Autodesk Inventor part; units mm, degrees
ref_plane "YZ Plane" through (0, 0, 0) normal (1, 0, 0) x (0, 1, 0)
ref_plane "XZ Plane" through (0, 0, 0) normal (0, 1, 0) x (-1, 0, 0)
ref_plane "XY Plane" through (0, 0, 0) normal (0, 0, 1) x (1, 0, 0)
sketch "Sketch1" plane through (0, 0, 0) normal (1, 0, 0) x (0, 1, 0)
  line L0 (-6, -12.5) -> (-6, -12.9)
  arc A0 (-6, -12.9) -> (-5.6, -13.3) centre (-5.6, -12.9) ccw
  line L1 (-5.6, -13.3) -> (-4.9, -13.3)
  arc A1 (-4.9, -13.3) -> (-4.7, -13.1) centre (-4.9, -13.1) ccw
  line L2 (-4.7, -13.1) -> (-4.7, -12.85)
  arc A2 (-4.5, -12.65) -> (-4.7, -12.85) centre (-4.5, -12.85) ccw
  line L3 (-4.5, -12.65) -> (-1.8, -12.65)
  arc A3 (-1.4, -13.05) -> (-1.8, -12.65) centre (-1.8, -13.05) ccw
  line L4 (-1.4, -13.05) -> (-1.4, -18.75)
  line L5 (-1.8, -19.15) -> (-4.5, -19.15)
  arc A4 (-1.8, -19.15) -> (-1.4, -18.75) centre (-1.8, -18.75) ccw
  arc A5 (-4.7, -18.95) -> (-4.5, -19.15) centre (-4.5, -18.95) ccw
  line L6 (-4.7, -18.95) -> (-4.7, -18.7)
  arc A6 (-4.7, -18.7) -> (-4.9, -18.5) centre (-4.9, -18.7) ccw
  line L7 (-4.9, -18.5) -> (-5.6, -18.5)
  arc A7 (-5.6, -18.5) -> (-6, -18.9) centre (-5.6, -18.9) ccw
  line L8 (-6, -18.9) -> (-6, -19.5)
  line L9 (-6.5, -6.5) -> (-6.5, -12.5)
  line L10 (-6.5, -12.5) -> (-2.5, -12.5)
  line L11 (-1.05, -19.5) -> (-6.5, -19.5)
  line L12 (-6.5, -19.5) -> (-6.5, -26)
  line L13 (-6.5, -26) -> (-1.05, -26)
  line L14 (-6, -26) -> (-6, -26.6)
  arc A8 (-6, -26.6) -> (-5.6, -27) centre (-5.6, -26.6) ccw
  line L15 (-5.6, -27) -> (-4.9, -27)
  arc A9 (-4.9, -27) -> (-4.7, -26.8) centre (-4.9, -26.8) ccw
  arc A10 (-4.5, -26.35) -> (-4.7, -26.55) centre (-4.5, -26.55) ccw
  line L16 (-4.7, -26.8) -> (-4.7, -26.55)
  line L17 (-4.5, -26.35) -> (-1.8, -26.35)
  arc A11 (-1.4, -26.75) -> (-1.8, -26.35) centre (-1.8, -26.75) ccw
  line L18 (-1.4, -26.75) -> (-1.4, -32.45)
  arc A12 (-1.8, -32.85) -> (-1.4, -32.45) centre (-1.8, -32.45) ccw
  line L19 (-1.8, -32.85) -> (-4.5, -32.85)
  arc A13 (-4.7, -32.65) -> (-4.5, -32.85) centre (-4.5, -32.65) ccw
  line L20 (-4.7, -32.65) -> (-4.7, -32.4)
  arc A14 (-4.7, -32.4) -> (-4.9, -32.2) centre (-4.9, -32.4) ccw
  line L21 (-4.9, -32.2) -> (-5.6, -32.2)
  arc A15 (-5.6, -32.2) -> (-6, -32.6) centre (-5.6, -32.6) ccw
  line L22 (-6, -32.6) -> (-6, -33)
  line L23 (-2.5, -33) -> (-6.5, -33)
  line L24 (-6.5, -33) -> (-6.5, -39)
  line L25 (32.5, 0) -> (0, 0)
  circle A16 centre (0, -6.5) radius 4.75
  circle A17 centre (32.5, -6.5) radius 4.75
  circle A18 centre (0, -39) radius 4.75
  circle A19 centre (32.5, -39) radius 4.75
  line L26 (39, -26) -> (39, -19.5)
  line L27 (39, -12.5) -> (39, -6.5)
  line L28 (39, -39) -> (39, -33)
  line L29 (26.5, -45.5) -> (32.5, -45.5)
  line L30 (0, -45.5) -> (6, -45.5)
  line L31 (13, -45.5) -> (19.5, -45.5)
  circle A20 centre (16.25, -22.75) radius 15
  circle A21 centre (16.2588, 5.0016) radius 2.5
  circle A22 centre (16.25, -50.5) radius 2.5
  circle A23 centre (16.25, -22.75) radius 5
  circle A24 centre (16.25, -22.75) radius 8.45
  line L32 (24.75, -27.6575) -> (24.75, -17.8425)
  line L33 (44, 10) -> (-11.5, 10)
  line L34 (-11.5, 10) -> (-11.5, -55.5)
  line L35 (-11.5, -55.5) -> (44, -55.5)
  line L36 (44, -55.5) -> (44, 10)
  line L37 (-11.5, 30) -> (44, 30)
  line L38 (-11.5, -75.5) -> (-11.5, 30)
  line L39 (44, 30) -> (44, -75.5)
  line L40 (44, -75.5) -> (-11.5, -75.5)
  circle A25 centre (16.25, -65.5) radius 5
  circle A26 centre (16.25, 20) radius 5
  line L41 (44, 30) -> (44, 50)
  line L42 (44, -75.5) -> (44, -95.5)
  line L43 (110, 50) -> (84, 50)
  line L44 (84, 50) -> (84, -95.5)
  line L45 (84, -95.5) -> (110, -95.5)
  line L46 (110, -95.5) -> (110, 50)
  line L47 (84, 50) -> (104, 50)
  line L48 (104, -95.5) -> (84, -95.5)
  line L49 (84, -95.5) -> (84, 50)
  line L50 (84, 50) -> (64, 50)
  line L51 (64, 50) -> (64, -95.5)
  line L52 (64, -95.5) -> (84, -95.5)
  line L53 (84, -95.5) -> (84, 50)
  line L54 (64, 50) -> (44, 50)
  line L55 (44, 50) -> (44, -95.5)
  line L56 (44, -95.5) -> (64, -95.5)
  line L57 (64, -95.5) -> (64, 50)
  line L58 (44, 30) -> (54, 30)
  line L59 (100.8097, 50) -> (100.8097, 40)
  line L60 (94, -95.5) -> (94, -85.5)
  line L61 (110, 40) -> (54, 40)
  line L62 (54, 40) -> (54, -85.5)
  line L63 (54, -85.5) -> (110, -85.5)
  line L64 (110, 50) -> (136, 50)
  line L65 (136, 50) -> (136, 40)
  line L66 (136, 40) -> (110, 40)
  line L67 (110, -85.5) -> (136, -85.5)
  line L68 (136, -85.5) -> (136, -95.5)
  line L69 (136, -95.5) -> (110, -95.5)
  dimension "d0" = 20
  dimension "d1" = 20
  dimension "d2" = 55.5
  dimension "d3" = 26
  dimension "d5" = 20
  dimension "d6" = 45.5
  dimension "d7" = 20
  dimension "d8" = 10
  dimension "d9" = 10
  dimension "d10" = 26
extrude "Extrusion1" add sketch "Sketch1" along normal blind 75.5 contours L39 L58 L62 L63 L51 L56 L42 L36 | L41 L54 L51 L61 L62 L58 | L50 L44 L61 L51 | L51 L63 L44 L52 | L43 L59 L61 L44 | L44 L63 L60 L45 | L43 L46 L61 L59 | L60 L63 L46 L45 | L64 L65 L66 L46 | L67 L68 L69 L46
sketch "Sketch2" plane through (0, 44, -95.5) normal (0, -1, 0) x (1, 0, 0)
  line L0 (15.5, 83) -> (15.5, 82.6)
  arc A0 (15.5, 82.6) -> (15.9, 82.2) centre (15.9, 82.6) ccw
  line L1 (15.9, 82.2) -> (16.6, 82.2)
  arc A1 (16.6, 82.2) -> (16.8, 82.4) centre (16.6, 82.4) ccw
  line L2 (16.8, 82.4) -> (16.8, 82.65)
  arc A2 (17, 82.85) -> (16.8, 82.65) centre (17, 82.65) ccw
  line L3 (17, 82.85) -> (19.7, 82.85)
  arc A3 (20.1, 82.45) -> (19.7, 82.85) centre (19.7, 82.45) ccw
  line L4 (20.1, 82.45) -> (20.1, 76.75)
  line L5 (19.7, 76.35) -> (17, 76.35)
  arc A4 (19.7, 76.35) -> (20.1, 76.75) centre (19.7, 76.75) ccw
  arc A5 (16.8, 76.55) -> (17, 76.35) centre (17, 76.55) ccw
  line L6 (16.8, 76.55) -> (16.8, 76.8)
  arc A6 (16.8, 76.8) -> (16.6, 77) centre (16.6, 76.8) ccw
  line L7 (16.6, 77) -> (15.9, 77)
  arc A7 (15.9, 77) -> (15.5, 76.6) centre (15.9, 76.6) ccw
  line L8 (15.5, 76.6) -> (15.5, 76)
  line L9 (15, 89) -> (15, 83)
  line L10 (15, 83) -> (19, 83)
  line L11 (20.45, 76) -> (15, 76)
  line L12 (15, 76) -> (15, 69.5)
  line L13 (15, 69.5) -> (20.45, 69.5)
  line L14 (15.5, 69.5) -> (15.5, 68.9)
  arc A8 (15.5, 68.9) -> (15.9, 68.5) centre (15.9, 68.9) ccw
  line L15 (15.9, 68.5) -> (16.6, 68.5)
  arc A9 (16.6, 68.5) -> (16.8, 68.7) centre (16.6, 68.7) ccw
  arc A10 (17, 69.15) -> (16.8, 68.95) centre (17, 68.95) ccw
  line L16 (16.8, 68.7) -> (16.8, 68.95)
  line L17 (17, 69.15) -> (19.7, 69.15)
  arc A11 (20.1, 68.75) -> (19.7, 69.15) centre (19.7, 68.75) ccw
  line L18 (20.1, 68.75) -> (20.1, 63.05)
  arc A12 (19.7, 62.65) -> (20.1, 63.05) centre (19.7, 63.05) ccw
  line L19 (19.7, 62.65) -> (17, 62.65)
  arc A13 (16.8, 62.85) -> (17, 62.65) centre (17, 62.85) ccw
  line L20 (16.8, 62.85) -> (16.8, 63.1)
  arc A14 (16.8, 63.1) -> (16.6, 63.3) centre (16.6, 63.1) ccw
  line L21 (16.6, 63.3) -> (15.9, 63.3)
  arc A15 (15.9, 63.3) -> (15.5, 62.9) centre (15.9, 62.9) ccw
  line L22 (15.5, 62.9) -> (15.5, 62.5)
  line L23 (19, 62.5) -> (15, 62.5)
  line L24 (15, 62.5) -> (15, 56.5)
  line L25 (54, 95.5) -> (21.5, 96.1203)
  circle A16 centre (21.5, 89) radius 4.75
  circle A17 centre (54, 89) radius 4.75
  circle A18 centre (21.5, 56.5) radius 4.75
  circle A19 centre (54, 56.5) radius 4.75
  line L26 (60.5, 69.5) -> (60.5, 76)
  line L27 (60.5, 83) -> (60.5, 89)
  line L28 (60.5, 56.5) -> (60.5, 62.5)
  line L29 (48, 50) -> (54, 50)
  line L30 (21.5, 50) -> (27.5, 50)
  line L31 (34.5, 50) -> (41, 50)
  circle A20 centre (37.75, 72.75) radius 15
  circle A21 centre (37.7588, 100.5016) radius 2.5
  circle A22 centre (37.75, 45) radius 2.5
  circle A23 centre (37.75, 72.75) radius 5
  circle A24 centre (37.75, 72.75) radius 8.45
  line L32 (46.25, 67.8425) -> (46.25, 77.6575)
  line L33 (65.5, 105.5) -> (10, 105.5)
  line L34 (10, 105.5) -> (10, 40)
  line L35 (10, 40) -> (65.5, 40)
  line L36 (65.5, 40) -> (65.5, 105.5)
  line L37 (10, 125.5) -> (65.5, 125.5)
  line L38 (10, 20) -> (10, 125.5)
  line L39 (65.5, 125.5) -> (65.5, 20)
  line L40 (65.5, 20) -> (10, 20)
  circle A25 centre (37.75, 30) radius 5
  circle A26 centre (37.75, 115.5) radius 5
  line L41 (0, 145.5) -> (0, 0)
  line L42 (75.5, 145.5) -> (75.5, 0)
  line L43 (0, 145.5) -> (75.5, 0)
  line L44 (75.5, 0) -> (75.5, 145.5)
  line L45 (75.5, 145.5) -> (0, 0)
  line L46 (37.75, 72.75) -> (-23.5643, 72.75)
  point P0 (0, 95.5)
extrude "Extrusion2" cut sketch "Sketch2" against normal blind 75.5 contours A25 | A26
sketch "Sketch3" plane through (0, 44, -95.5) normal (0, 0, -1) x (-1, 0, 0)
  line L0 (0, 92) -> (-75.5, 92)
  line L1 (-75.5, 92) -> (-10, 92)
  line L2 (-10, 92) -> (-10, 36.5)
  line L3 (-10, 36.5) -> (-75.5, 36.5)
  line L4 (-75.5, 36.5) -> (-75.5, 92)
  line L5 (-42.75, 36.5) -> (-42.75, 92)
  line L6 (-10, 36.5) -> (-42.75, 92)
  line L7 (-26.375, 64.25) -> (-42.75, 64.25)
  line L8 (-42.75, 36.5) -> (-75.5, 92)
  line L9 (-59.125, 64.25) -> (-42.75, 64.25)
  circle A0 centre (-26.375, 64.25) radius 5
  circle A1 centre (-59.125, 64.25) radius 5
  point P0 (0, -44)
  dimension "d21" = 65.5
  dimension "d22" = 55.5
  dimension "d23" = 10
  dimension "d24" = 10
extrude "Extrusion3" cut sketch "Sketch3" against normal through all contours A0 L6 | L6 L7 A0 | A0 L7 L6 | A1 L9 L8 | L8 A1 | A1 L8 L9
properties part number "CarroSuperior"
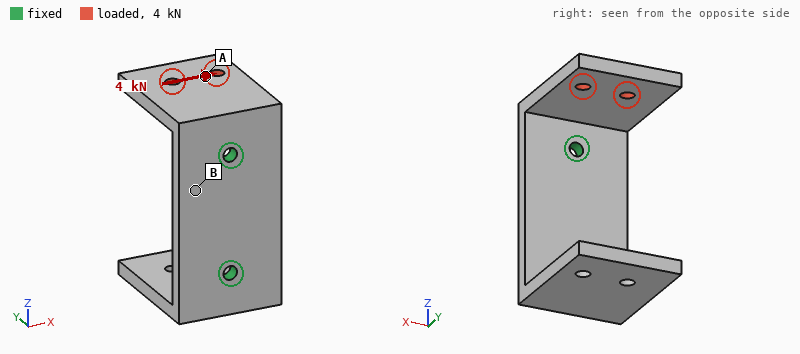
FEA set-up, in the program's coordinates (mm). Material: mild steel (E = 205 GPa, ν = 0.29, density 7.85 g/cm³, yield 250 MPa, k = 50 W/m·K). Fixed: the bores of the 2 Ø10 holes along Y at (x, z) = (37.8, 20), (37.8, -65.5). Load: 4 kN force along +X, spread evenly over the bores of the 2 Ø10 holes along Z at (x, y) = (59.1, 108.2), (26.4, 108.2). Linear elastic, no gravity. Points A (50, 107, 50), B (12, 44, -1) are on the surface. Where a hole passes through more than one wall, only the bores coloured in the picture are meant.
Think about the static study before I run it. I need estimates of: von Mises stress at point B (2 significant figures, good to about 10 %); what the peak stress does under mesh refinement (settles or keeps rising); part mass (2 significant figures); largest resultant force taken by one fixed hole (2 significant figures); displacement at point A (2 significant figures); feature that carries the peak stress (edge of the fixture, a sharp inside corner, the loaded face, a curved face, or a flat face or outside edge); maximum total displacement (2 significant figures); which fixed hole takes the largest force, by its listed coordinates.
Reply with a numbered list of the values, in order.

1. 54 MPa
2. keeps rising
3. 1.8 kg
4. 4.9 kN
5. 0.17 mm
6. edge of the fixture
7. 0.28 mm
8. (37.8, 20)
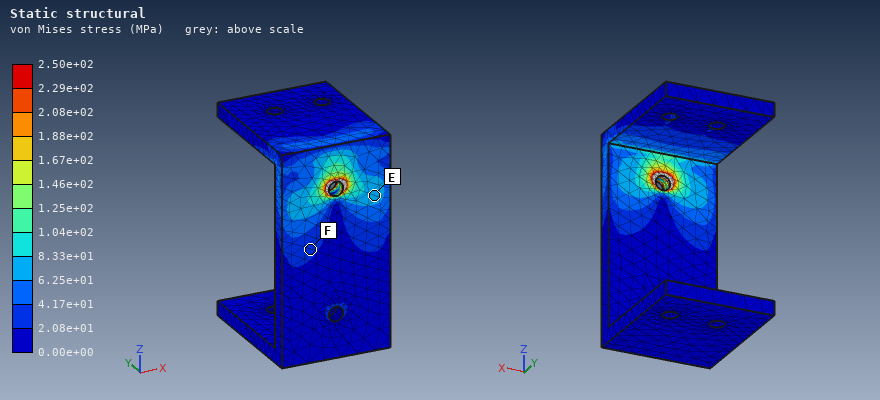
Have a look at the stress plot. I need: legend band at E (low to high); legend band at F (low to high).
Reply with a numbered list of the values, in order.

1. 6.25e+01 to 8.33e+01 MPa
2. 2.08e+01 to 4.17e+01 MPa
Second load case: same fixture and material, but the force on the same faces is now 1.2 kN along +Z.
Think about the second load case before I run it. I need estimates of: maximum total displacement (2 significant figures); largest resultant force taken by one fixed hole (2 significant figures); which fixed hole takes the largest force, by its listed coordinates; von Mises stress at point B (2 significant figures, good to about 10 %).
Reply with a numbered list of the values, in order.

1. 0.23 mm
2. 1.1 kN
3. (37.8, 20)
4. 9.0 MPa
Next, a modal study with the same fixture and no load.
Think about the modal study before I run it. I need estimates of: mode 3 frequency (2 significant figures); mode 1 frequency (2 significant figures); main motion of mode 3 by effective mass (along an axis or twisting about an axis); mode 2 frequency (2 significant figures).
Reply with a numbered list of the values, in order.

1. 1100 Hz
2. 750 Hz
3. along X
4. 760 Hz
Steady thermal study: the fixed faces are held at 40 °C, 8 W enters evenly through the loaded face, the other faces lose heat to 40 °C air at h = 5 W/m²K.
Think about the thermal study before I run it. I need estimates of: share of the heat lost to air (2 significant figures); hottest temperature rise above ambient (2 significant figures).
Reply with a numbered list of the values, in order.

1. 15 %
2. 19 K
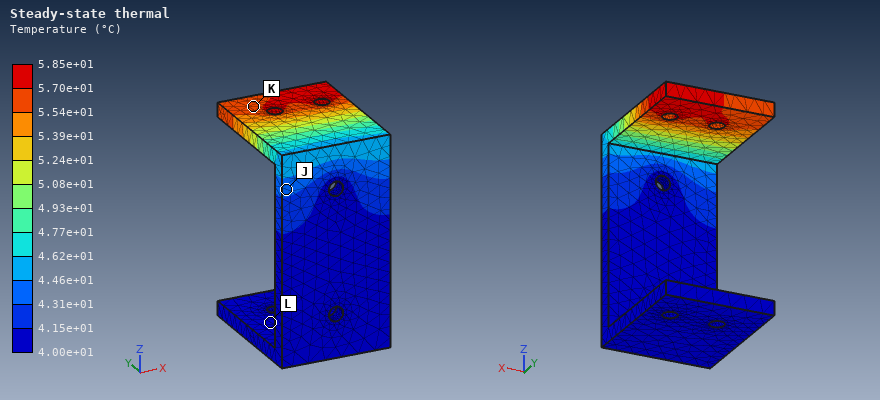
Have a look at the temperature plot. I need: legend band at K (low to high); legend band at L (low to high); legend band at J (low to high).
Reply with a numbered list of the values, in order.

1. 5.54e+01 to 5.70e+01 °C
2. 4.00e+01 to 4.15e+01 °C
3. 4.31e+01 to 4.46e+01 °C
